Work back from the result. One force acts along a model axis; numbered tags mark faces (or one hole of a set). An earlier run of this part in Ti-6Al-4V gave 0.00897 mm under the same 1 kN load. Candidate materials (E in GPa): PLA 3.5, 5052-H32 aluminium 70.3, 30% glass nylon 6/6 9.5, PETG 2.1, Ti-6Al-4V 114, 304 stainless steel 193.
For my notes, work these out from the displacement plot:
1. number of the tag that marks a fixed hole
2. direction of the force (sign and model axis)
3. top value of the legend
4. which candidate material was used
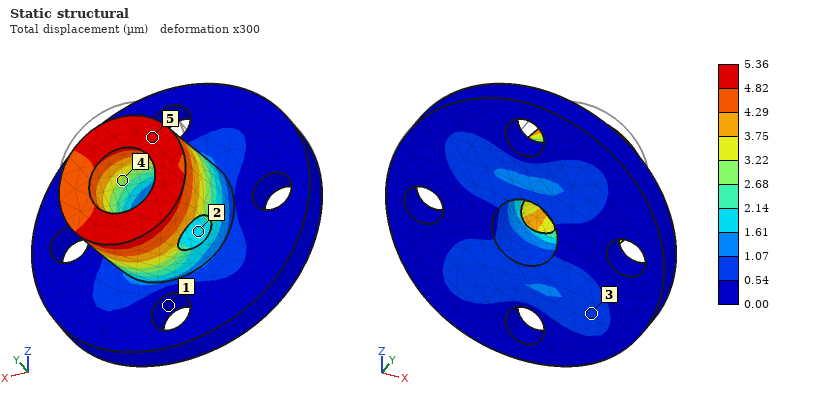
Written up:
1
-Z
5.36 µm
304 stainless steel
